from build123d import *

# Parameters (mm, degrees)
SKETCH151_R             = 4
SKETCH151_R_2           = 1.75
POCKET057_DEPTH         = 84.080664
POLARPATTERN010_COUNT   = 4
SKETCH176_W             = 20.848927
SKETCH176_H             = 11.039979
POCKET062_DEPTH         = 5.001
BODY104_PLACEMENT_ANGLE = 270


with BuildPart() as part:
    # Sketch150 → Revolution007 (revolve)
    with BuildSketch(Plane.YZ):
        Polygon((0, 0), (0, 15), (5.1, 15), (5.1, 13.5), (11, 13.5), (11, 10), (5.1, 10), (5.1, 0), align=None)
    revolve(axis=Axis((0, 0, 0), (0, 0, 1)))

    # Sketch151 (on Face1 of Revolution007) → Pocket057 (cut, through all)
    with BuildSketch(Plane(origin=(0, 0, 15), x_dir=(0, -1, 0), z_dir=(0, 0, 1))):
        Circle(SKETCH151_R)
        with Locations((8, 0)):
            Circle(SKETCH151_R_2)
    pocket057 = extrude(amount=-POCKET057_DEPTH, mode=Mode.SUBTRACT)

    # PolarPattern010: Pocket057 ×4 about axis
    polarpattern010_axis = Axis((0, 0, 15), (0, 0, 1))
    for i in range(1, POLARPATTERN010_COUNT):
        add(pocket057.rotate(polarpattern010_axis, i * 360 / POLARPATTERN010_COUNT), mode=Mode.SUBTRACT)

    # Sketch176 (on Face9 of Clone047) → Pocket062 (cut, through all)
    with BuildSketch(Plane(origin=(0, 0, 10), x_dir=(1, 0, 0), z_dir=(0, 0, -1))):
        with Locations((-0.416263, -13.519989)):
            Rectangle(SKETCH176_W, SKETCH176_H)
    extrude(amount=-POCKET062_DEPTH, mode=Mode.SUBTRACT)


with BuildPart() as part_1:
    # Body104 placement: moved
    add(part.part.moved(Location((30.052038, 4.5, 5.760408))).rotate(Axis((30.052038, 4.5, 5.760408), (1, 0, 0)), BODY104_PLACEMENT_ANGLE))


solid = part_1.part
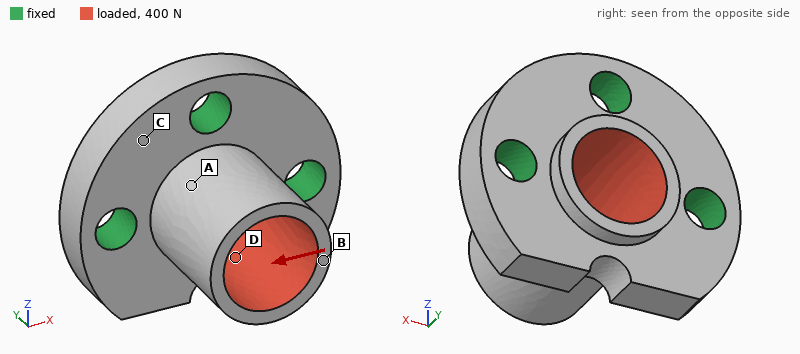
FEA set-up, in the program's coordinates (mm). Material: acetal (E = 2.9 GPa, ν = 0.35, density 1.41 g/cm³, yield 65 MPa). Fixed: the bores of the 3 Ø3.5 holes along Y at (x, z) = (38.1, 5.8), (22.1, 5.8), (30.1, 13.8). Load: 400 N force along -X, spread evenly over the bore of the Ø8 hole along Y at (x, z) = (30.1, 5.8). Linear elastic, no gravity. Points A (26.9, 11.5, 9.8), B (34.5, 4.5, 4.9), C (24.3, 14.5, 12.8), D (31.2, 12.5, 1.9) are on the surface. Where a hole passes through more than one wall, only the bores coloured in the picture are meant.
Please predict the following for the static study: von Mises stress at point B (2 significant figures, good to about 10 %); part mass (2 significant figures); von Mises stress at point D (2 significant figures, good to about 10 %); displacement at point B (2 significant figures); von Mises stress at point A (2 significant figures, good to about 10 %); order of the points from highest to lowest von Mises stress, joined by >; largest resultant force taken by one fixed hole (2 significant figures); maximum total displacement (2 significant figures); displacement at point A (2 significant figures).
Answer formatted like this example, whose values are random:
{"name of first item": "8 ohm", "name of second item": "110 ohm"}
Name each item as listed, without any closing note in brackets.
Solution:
{"von Mises stress at point B": "5.5 MPa", "part mass": "1.8 g", "von Mises stress at point D": "24 MPa", "displacement at point B": "0.17 mm", "von Mises stress at point A": "14 MPa", "order of the points from highest to lowest von Mises stress, joined by >": "D > A > B > C", "largest resultant force taken by one fixed hole": "210 N", "maximum total displacement": "0.17 mm", "displacement at point A": "0.068 mm"}
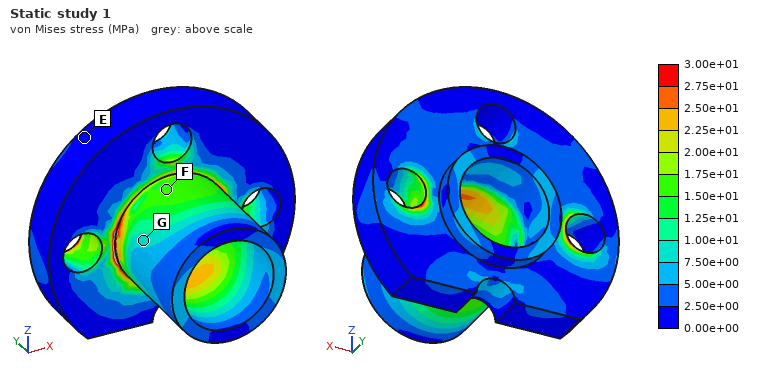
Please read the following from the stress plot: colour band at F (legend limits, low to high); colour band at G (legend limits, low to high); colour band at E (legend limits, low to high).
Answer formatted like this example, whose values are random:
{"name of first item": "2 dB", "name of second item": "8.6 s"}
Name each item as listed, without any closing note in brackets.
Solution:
{"colour band at F": "1.50e+01 to 1.75e+01 MPa", "colour band at G": "7.50e+00 to 1.00e+01 MPa", "colour band at E": "0.00e+00 to 2.50e+00 MPa"}
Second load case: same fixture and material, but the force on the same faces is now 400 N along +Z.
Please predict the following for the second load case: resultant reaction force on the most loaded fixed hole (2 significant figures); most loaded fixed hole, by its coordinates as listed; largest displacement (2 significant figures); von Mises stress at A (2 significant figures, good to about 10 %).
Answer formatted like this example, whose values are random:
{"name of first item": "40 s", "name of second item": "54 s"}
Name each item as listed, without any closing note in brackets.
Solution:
{"resultant reaction force on the most loaded fixed hole": "200 N", "most loaded fixed hole, by its coordinates as listed": "(30.1, 13.8)", "largest displacement": "0.28 mm", "von Mises stress at A": "15 MPa"}
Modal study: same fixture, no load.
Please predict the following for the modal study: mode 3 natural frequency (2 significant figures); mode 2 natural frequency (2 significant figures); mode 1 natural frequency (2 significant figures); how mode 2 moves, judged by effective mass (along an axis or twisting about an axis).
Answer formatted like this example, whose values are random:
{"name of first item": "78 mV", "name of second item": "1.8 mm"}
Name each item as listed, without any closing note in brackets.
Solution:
{"mode 3 natural frequency": "12 kHz", "mode 2 natural frequency": "11 kHz", "mode 1 natural frequency": "8000 Hz", "how mode 2 moves, judged by effective mass": "along X"}
